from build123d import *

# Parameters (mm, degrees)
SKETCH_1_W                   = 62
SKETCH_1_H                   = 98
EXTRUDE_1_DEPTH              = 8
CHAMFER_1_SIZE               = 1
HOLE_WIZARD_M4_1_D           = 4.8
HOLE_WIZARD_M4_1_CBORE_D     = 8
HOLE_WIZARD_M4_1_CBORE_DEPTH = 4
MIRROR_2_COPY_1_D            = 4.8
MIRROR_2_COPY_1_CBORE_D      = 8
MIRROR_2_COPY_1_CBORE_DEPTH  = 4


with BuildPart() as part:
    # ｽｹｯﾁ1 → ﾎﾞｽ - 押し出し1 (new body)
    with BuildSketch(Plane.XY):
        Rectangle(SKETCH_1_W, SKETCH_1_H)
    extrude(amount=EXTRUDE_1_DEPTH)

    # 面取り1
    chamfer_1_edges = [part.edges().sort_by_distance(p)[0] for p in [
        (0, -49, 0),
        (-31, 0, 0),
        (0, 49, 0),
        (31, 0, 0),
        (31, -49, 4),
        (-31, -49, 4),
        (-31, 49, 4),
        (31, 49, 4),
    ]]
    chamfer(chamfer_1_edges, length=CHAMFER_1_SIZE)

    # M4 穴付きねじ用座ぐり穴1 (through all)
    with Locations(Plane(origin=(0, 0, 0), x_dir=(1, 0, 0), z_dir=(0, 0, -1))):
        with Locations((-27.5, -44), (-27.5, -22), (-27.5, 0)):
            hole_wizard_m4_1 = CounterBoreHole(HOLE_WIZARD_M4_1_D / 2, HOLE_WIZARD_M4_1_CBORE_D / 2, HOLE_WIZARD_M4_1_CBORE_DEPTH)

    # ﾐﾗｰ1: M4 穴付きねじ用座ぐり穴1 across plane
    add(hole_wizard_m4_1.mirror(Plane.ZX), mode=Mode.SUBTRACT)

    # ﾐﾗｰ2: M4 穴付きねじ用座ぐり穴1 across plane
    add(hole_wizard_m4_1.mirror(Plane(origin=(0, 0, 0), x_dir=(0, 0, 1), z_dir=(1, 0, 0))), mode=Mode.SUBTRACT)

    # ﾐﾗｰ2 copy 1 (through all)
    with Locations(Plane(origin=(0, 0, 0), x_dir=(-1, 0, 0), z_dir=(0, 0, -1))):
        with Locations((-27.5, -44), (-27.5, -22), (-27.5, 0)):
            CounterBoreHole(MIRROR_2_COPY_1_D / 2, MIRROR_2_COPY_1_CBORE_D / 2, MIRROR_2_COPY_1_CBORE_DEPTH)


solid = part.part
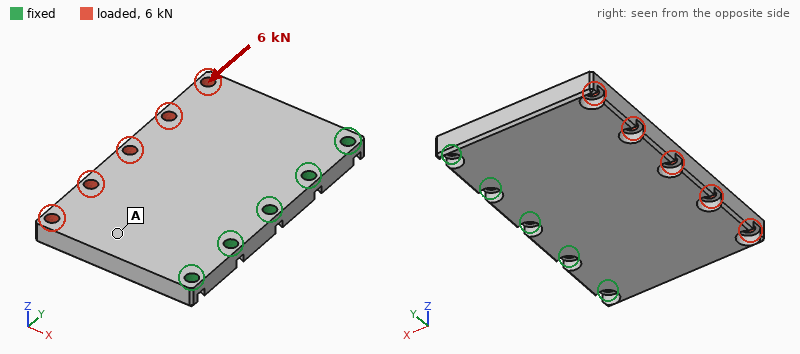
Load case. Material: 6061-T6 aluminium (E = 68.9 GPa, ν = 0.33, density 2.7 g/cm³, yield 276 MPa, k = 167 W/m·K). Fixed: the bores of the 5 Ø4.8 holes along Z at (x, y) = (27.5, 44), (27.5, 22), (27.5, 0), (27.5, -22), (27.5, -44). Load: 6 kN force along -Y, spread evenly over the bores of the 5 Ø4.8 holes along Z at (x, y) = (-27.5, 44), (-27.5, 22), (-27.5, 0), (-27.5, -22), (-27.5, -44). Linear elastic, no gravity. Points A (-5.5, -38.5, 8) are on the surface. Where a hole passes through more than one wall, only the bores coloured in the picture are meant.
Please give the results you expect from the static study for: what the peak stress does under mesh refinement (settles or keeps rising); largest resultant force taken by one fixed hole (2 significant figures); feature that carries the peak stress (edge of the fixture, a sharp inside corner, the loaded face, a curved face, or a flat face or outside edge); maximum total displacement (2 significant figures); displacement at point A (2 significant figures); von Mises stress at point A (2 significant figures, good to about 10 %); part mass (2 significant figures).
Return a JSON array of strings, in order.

["keeps rising", "3.2 kN", "edge of the fixture", "0.10 mm", "0.049 mm", "21 MPa", "120 g"]
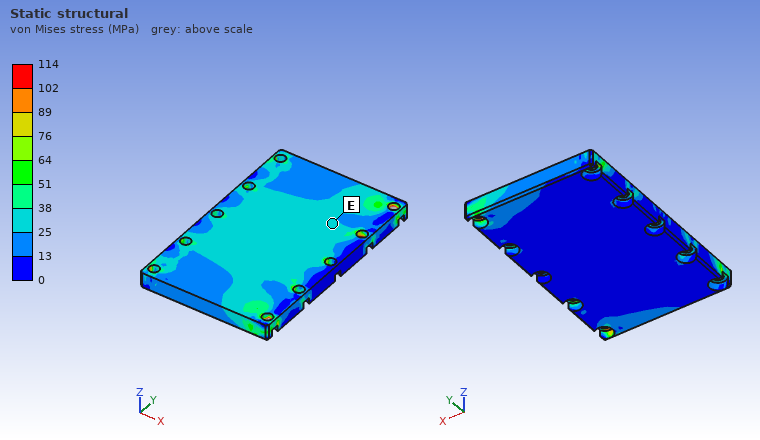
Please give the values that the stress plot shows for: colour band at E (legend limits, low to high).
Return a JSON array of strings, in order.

["25 to 38 MPa"]
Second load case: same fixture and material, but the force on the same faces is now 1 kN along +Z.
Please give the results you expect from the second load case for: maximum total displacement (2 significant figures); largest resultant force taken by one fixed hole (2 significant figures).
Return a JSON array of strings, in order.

["0.39 mm", "350 N"]
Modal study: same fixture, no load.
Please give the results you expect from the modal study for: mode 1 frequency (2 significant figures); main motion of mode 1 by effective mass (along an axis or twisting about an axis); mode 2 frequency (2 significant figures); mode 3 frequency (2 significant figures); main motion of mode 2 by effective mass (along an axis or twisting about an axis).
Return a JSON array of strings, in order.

["1400 Hz", "along Z", "2800 Hz", "6300 Hz", "twisting about X"]
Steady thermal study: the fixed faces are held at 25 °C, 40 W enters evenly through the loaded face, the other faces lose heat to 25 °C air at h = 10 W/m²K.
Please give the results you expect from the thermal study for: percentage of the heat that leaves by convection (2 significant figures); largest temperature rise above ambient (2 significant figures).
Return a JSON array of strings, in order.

["3.6 %", "24 K"]
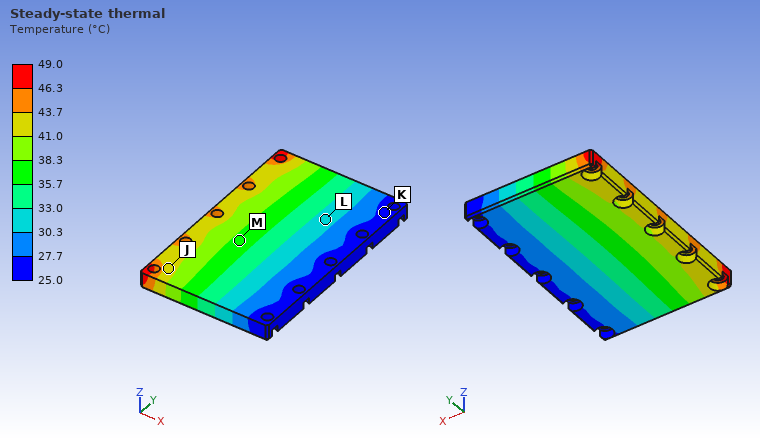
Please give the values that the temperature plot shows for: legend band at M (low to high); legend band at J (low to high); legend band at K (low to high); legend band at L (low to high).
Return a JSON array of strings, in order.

["35.7 to 38.3 °C", "41.0 to 43.7 °C", "25.0 to 27.7 °C", "30.3 to 33.0 °C"]
